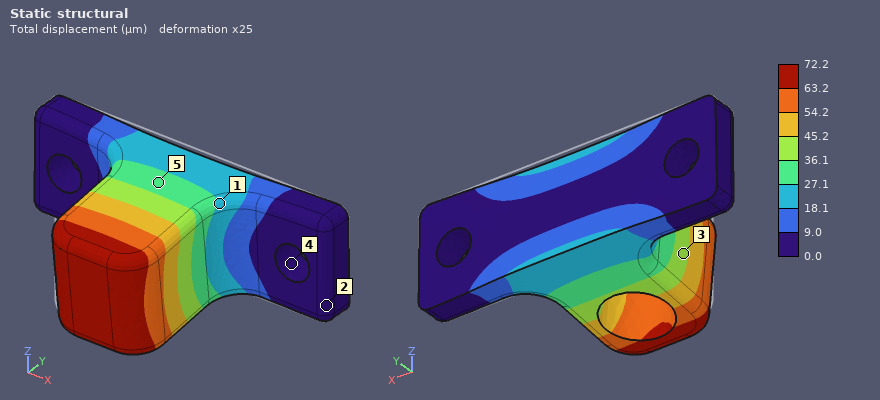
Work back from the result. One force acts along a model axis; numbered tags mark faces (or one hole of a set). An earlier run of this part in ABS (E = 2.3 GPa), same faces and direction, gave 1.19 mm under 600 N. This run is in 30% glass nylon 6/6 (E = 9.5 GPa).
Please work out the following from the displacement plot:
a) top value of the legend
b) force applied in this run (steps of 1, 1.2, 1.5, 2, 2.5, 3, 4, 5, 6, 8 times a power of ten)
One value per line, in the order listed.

72.2 µm
150 N
